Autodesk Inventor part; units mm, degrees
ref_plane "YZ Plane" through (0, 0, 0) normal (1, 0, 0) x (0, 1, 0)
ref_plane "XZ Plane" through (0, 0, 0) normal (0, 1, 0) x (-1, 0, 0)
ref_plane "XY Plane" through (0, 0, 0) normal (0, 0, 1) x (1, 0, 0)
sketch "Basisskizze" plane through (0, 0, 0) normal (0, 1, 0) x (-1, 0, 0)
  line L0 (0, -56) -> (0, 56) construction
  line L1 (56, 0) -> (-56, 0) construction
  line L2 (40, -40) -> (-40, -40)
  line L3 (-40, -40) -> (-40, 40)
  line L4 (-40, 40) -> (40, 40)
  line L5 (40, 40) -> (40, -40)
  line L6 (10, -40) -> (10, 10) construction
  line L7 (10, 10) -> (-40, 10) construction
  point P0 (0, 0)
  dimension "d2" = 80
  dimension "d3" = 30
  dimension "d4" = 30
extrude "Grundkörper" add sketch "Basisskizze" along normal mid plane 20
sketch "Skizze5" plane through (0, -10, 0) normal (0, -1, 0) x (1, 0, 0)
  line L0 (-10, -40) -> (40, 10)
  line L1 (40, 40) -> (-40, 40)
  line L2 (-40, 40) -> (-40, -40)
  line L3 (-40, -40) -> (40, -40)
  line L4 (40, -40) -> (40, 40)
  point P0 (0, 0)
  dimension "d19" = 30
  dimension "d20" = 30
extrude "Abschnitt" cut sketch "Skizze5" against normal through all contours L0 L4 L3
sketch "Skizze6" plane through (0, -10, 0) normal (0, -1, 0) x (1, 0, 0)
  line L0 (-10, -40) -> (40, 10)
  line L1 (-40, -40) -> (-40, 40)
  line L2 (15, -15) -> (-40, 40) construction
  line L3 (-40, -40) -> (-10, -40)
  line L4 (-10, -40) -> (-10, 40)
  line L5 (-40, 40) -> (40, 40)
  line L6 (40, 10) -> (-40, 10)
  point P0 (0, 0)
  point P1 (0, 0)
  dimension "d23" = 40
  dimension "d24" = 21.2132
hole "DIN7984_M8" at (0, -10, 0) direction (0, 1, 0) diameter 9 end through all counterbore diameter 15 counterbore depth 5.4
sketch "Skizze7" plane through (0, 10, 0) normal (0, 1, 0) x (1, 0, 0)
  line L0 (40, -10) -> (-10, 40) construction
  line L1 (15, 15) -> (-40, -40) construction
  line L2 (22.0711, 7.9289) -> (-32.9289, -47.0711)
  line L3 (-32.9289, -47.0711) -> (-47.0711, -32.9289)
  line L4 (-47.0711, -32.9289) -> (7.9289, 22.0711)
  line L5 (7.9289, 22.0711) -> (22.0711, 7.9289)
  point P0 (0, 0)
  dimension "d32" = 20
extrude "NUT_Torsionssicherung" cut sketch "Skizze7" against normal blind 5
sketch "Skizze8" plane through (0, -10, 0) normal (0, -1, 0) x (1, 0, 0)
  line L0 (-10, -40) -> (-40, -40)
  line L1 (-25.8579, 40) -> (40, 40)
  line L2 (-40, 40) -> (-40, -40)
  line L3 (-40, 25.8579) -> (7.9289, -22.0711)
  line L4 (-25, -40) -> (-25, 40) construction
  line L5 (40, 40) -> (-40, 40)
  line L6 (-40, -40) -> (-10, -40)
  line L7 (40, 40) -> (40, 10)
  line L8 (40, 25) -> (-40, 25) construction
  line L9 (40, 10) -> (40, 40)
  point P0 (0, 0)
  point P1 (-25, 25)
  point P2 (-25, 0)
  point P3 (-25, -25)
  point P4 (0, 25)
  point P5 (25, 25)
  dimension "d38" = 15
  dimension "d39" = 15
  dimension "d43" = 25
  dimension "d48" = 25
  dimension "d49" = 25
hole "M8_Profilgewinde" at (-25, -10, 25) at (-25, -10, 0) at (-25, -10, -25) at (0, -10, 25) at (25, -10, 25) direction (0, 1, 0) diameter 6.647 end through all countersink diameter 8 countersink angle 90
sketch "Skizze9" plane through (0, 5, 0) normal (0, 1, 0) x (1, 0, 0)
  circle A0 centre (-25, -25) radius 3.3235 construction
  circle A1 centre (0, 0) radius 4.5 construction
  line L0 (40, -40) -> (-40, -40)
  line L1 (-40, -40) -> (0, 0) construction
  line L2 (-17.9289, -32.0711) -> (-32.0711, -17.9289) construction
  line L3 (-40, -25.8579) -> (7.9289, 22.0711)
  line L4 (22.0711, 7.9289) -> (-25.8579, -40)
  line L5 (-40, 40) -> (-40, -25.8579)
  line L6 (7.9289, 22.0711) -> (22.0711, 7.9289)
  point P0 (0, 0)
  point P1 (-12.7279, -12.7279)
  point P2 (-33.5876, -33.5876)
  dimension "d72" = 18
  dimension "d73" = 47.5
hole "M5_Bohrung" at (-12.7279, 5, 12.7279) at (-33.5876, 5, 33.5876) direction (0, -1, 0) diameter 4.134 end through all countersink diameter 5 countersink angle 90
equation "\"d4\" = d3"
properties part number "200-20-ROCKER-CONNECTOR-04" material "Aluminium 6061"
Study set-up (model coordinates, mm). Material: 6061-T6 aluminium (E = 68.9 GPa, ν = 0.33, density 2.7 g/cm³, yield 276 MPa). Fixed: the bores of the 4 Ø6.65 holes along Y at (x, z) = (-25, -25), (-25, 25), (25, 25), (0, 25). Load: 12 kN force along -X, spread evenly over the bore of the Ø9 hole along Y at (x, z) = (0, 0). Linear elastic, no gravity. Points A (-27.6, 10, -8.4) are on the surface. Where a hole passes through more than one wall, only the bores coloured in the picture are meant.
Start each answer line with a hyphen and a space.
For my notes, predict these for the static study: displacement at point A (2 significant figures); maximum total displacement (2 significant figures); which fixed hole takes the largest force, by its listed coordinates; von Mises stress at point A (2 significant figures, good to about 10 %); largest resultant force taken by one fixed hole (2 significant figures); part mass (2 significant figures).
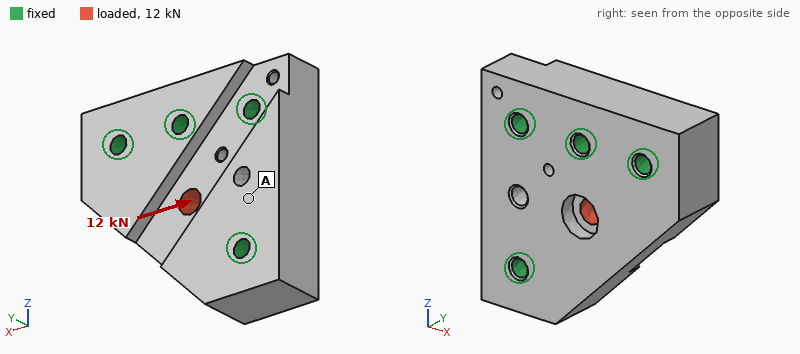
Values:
- 4.1 µm
- 12 µm
- (-25, -25)
- 6.4 MPa
- 4.7 kN
- 240 g
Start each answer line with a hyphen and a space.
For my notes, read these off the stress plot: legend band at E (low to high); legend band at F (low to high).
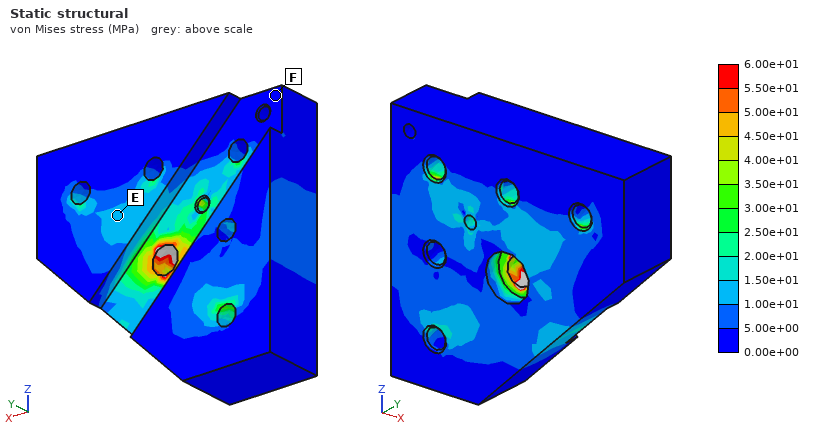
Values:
- 1.00e+01 to 1.50e+01 MPa
- 0.00e+00 to 5.00e+00 MPa
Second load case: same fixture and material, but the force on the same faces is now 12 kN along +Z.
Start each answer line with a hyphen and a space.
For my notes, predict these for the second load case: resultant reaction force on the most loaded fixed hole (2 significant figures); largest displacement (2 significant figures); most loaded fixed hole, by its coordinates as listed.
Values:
- 5.0 kN
- 12 µm
- (0, 25)
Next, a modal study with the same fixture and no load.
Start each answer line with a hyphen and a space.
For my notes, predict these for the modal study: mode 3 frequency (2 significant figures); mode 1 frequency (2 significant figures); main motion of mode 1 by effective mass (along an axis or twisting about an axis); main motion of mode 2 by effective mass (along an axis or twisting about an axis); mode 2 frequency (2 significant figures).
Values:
- 23 kHz
- 14 kHz
- along Y
- along Y
- 20 kHz
